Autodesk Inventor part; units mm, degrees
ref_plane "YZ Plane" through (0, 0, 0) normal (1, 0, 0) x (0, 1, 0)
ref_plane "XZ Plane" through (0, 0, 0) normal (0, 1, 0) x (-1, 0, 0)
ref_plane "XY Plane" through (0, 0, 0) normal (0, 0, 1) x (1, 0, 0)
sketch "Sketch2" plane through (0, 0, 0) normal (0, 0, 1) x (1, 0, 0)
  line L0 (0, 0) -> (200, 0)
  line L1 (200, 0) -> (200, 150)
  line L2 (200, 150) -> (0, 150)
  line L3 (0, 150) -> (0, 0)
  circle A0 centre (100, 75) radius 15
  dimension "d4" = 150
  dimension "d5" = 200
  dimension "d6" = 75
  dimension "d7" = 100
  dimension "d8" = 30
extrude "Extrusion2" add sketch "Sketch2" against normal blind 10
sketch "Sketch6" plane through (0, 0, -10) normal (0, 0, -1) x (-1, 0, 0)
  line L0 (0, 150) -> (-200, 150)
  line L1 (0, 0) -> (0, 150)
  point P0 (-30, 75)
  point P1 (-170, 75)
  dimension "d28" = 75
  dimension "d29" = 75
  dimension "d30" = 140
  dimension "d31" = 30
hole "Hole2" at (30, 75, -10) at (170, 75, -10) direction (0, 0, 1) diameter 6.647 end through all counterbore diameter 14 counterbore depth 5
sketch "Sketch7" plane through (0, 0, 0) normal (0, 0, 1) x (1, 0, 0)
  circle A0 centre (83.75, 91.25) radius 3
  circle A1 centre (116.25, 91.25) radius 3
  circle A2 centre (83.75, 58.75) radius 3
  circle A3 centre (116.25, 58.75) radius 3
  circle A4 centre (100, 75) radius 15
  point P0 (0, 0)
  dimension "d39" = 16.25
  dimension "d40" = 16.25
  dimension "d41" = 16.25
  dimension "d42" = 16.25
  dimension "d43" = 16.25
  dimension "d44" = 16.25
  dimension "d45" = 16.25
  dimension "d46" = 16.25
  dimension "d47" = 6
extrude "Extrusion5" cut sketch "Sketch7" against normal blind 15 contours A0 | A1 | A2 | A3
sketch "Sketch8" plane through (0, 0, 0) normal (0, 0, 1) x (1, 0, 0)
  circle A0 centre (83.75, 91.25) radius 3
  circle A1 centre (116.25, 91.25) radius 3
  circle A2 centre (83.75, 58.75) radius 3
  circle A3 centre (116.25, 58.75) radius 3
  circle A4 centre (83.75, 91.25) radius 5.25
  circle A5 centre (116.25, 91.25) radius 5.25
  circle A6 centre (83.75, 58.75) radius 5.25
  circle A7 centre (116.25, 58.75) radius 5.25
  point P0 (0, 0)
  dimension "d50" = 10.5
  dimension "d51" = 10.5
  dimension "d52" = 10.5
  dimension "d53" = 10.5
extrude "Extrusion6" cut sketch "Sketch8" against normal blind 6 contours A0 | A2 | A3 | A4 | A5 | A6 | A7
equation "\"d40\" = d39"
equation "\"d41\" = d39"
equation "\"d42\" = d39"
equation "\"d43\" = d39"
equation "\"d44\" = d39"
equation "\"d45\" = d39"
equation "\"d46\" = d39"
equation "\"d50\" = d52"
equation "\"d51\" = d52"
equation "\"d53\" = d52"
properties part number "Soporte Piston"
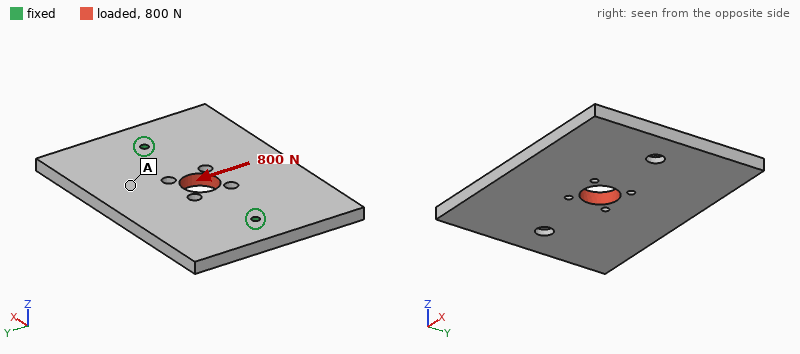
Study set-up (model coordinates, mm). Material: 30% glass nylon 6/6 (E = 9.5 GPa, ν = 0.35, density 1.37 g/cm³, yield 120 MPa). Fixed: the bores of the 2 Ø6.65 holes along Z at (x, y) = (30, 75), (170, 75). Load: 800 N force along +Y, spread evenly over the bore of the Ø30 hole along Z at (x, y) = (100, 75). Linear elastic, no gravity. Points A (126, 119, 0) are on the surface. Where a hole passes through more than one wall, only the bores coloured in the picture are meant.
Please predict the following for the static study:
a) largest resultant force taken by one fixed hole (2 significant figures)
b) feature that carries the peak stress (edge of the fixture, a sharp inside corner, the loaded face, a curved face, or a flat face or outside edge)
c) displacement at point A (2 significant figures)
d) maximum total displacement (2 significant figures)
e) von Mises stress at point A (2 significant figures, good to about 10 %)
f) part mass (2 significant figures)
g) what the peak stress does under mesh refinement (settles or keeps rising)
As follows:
400 N
edge of the fixture
37 µm
65 µm
0.54 MPa
400 g
keeps rising
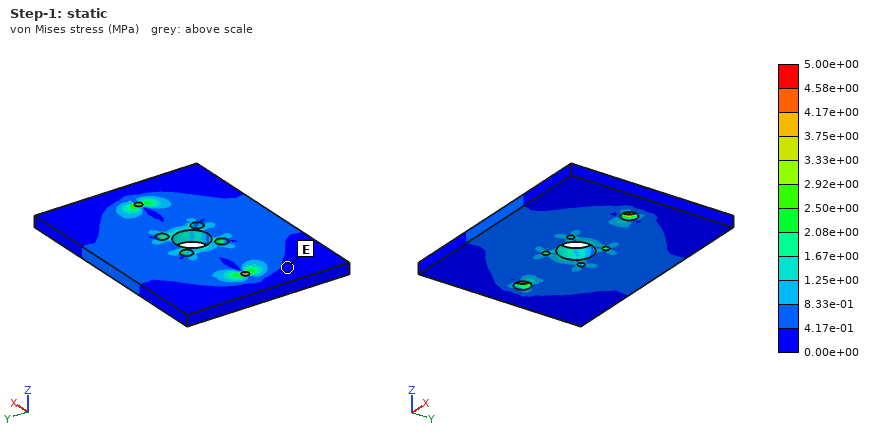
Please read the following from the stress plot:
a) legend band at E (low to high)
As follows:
0.00e+00 to 4.17e-01 MPa
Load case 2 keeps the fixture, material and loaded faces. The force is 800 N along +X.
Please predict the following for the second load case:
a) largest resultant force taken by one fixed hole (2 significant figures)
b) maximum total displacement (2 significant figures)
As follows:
400 N
10 µm
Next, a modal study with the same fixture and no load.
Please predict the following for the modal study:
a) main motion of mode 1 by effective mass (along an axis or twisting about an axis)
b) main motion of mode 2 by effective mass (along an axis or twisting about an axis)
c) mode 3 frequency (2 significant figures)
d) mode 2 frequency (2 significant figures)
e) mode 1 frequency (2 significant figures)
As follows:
twisting about X
along Z
630 Hz
560 Hz
270 Hz
